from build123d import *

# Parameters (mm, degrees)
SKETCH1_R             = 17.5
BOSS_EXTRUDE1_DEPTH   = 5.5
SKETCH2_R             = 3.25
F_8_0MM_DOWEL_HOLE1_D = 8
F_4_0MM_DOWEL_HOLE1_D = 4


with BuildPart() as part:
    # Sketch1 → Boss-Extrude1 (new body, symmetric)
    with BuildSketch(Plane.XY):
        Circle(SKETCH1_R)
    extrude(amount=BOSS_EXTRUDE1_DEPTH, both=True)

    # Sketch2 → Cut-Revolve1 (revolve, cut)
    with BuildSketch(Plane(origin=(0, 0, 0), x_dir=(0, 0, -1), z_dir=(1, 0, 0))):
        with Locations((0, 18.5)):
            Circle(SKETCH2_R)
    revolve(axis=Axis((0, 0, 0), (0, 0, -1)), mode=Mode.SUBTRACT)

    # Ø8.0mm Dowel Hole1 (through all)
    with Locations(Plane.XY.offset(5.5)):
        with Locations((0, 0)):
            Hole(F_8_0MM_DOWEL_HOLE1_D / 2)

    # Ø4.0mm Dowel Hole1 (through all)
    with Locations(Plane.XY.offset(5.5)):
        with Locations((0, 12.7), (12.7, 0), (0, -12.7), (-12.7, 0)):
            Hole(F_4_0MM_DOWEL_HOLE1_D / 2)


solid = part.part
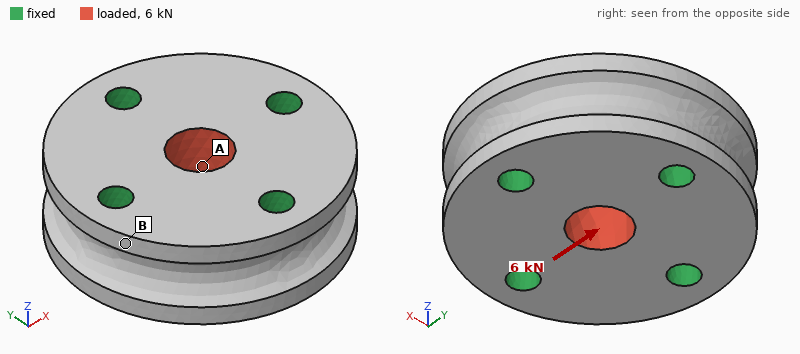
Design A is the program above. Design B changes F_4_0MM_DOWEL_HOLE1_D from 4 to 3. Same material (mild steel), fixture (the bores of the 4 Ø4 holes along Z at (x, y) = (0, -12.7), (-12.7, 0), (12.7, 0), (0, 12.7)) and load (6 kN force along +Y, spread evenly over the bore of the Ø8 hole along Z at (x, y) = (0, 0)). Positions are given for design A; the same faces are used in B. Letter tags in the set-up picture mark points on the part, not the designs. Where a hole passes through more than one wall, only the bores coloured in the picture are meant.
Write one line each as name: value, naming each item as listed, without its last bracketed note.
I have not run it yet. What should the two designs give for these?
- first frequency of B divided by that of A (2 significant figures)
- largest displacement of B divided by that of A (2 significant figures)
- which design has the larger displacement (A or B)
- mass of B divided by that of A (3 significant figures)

first frequency of B divided by that of A: 0.92
largest displacement of B divided by that of A: 1.1
which design has the larger displacement: B
mass of B divided by that of A: 1.03
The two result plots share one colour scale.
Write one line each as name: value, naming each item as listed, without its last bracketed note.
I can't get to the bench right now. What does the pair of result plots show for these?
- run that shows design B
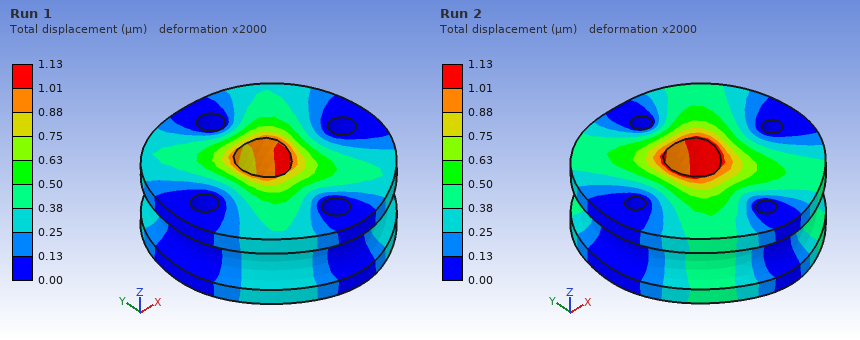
run that shows design B: Run 2
